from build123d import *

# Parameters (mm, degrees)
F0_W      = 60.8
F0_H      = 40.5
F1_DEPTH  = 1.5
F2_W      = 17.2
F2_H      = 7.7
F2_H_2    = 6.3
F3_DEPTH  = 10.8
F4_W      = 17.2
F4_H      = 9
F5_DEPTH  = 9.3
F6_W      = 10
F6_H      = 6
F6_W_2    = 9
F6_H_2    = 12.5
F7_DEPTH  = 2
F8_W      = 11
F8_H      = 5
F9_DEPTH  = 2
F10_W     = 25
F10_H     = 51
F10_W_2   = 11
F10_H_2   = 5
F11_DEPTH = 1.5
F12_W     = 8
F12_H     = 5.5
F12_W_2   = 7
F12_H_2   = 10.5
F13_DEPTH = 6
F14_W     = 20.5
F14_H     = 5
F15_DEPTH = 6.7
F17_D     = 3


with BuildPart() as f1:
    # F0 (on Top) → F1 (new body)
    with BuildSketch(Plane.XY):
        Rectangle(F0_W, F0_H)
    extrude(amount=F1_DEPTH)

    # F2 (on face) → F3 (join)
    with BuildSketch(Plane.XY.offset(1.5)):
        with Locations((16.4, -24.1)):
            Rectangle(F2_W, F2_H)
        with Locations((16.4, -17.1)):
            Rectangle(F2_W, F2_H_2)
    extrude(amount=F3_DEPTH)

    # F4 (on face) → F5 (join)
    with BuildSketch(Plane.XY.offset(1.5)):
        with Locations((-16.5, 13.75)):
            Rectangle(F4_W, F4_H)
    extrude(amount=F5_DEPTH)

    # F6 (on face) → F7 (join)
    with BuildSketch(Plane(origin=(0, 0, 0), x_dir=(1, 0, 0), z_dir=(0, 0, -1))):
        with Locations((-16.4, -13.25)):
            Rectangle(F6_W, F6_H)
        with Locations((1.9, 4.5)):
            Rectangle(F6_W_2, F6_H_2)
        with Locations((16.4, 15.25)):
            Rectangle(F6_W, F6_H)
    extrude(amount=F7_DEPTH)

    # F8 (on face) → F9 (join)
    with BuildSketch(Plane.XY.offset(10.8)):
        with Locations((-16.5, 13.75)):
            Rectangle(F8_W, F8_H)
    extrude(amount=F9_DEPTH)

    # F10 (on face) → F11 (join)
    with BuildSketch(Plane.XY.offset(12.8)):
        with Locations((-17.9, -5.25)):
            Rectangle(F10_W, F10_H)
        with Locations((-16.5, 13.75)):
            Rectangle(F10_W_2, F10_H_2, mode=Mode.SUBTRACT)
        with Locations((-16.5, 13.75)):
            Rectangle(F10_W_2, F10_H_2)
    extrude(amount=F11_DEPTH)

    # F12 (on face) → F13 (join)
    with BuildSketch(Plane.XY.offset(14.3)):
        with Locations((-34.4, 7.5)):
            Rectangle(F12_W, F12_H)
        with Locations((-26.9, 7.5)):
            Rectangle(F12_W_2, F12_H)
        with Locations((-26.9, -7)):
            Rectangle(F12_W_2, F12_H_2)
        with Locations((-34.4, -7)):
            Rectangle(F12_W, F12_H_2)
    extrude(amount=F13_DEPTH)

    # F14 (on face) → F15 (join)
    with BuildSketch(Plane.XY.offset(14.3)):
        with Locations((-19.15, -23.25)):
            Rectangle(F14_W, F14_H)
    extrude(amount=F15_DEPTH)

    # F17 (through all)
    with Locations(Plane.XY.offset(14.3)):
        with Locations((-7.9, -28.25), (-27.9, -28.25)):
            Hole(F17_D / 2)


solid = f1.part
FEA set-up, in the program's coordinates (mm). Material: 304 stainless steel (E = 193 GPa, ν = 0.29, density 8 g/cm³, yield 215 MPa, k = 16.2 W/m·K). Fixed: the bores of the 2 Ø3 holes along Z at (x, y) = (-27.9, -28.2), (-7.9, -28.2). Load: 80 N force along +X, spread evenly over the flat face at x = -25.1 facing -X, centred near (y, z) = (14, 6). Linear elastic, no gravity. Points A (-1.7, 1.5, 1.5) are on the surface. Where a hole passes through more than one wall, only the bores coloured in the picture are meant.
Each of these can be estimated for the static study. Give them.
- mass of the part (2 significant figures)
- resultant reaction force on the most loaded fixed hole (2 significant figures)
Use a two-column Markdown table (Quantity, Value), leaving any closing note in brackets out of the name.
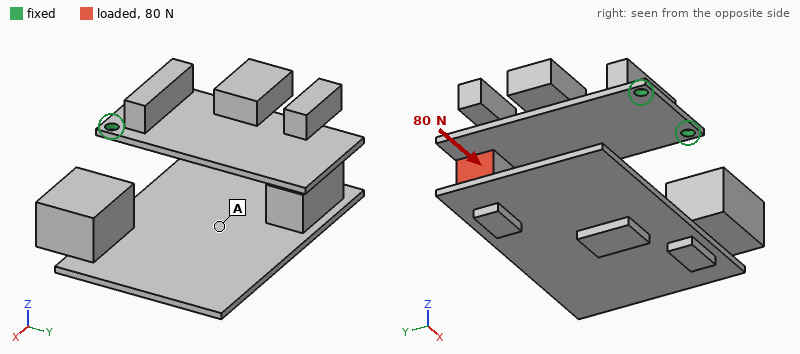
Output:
| Quantity | Value |
|---|---|
| mass of the part | 99 g |
| resultant reaction force on the most loaded fixed hole | 170 N |
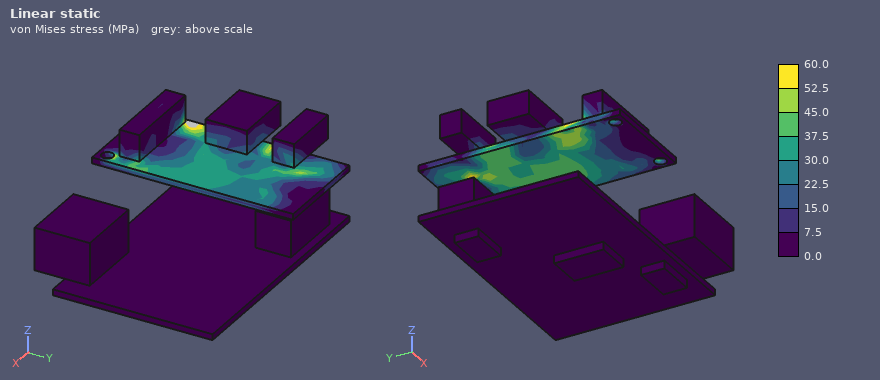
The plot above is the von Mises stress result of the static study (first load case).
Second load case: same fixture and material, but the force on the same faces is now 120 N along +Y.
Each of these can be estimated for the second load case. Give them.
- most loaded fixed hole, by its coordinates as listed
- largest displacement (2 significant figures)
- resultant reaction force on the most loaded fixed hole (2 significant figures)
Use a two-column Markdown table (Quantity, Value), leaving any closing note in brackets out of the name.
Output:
| Quantity | Value |
|---|---|
| most loaded fixed hole, by its coordinates as listed | (-27.9, -28.2) |
| largest displacement | 0.58 mm |
| resultant reaction force on the most loaded fixed hole | 110 N |
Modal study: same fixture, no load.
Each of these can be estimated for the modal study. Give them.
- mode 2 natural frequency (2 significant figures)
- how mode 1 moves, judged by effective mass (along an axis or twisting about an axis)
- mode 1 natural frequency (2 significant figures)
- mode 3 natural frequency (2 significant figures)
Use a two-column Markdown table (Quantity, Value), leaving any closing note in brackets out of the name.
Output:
| Quantity | Value |
|---|---|
| mode 2 natural frequency | 210 Hz |
| how mode 1 moves, judged by effective mass | along Z |
| mode 1 natural frequency | 170 Hz |
| mode 3 natural frequency | 500 Hz |
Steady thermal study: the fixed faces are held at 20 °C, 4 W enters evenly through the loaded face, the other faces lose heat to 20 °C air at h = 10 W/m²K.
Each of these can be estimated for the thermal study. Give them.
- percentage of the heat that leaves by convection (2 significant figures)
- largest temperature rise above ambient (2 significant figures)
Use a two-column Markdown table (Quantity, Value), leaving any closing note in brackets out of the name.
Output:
| Quantity | Value |
|---|---|
| percentage of the heat that leaves by convection | 84 % |
| largest temperature rise above ambient | 80 K |
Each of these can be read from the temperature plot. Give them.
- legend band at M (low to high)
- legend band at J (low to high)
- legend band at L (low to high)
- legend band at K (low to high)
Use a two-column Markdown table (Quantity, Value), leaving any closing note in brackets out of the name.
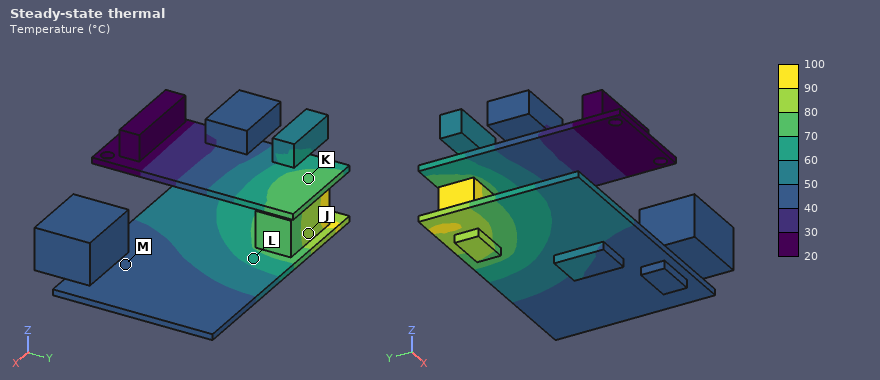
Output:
| Quantity | Value |
|---|---|
| legend band at M | 40 to 50 °C |
| legend band at J | 80 to 90 °C |
| legend band at L | 60 to 70 °C |
| legend band at K | 70 to 80 °C |
